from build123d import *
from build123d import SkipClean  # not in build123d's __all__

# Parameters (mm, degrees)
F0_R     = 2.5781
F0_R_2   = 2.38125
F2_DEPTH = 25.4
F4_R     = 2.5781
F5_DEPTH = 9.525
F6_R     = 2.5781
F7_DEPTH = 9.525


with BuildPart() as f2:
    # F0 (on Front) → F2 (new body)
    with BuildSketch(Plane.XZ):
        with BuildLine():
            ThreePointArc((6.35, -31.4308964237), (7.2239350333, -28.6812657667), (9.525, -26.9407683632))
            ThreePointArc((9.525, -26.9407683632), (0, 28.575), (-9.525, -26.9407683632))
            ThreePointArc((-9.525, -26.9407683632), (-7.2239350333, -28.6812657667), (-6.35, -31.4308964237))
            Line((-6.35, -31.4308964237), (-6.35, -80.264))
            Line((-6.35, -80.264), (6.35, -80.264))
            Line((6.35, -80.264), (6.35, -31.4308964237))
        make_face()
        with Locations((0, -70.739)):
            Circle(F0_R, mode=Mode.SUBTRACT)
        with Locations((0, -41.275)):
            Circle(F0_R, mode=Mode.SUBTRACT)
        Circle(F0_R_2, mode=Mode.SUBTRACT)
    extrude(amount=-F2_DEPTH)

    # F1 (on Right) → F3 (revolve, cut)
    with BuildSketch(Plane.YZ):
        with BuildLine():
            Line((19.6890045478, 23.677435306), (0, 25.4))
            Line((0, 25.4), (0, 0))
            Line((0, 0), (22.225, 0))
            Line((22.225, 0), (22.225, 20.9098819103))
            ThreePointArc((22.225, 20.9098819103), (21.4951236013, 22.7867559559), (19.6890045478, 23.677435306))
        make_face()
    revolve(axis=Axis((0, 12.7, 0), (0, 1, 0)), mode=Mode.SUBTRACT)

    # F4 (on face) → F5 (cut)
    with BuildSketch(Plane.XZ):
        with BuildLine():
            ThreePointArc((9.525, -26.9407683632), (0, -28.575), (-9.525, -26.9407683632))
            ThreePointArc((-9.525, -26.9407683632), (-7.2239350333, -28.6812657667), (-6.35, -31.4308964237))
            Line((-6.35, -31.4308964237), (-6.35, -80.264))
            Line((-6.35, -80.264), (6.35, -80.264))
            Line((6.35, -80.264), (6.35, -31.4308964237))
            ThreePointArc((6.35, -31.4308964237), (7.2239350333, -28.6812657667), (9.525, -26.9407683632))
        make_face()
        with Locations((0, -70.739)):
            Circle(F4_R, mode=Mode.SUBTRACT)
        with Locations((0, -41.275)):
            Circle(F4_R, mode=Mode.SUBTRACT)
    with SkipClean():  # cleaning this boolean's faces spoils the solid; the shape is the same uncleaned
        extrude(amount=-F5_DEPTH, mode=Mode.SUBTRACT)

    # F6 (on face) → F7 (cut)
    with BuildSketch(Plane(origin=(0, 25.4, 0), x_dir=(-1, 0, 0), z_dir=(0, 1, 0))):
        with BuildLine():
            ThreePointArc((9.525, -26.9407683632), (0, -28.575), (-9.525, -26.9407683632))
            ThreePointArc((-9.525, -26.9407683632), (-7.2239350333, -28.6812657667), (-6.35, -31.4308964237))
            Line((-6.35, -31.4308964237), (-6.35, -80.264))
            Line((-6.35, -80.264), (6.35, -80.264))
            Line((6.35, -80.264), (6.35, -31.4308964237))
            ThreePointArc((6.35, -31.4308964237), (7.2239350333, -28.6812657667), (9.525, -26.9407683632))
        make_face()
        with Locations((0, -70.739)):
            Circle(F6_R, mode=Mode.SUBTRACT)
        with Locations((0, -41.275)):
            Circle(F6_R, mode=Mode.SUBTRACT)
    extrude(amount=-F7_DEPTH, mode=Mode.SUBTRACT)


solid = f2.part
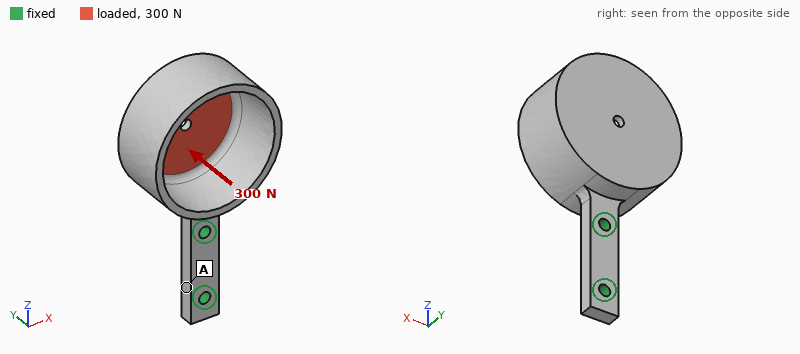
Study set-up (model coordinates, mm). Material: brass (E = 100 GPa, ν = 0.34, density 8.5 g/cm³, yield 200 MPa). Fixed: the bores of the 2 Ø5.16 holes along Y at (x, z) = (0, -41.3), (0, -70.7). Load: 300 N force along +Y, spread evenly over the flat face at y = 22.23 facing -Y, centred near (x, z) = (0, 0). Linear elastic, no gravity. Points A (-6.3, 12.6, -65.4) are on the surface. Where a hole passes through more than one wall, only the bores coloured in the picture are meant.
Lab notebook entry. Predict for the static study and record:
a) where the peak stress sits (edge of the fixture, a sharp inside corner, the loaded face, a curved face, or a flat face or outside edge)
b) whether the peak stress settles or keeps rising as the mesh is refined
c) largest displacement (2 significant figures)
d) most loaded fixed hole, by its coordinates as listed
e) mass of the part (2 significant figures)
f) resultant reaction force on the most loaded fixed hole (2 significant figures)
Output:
edge of the fixture
keeps rising
0.38 mm
(0, -41.3)
230 g
320 N
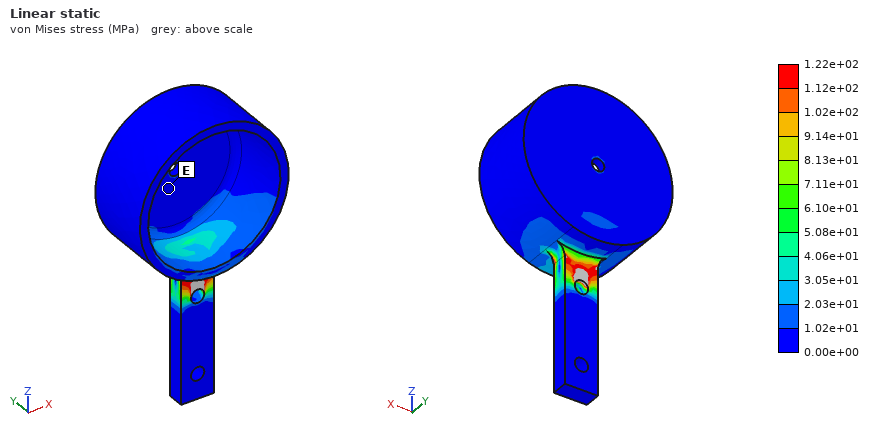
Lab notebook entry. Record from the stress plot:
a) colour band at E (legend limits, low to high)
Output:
0.00e+00 to 1.02e+01 MPa
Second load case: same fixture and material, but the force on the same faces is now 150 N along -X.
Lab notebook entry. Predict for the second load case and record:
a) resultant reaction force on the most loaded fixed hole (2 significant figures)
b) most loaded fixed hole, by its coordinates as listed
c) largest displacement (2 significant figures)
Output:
210 N
(0, -41.3)
80 µm
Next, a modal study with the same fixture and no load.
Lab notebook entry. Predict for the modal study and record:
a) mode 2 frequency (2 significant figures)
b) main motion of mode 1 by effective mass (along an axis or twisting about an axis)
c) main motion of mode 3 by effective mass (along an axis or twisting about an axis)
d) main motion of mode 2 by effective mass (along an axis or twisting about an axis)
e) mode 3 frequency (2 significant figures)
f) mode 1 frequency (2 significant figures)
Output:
540 Hz
along Y
twisting about Z
along X
870 Hz
380 Hz
